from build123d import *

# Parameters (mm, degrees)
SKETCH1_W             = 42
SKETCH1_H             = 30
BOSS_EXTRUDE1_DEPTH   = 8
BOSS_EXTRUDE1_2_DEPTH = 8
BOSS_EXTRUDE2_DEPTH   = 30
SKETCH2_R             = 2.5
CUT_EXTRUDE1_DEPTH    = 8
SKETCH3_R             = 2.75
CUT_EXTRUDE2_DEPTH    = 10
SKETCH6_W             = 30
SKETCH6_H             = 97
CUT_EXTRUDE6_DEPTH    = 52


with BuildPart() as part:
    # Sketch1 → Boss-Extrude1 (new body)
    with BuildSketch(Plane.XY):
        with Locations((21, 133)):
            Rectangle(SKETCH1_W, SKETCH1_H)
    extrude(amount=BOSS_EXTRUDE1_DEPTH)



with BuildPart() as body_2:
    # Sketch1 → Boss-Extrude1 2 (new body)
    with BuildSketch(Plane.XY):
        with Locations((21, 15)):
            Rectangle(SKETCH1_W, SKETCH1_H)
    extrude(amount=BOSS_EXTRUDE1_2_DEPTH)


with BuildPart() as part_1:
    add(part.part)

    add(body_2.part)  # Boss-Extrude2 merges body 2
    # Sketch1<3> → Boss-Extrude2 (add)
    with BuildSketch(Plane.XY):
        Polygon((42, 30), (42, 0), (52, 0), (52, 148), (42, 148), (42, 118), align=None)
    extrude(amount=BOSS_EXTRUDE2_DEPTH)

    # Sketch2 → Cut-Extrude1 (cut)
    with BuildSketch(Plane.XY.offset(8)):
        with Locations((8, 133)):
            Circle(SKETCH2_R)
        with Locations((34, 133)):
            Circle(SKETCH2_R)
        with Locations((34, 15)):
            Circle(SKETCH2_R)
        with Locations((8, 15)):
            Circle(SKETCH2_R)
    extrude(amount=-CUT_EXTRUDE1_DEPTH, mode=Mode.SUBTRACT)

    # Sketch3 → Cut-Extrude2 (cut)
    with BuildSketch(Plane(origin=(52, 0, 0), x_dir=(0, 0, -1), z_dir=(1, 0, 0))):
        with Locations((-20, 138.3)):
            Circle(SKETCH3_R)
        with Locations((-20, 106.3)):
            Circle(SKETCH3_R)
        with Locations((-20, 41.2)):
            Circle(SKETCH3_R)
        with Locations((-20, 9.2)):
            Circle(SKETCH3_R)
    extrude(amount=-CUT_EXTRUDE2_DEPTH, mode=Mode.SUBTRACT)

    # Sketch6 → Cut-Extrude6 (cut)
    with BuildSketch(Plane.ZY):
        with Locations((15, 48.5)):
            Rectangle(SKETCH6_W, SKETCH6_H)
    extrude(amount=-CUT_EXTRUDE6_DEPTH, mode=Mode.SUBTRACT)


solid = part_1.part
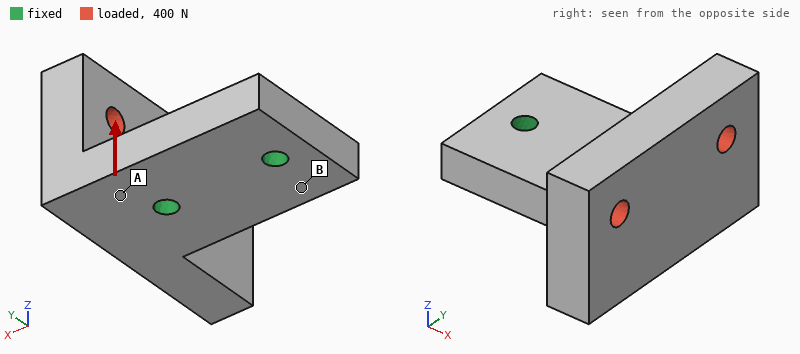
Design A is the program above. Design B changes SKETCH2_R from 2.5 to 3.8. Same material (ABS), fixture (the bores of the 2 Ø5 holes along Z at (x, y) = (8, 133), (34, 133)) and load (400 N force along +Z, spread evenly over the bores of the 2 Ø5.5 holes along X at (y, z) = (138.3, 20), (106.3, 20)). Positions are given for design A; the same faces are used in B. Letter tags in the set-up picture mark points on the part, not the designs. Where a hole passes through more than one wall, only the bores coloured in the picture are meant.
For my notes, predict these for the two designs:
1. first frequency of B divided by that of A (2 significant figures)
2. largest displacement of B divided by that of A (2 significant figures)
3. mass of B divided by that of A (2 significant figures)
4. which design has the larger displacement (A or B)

1.1
0.78
0.98
A
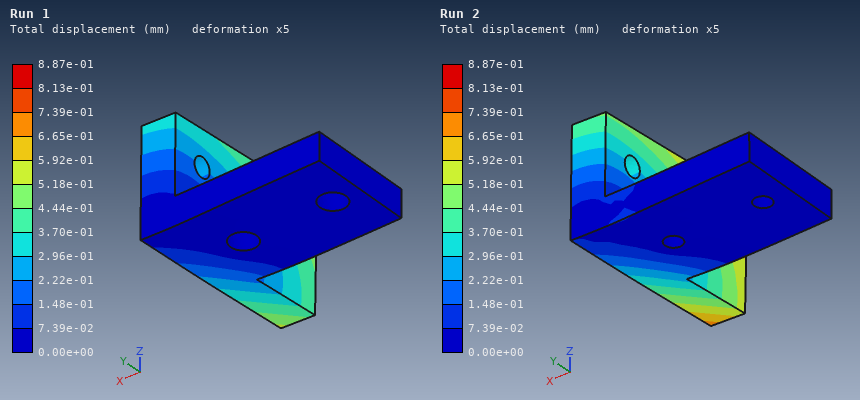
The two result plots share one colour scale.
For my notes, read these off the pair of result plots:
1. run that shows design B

Run 1
